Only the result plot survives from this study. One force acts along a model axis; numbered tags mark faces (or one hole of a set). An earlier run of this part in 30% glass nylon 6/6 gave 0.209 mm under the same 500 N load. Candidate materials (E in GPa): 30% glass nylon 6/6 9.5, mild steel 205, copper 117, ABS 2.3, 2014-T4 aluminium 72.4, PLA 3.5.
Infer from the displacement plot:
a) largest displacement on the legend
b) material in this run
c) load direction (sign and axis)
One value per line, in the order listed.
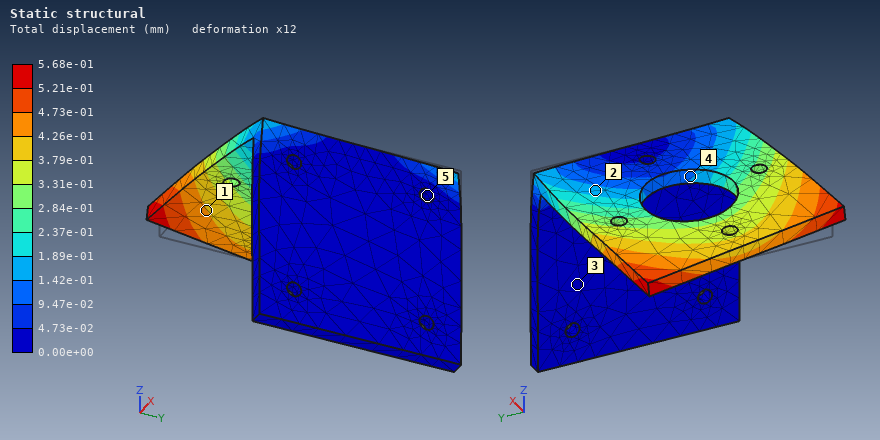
5.68e-01 mm
PLA
-Y
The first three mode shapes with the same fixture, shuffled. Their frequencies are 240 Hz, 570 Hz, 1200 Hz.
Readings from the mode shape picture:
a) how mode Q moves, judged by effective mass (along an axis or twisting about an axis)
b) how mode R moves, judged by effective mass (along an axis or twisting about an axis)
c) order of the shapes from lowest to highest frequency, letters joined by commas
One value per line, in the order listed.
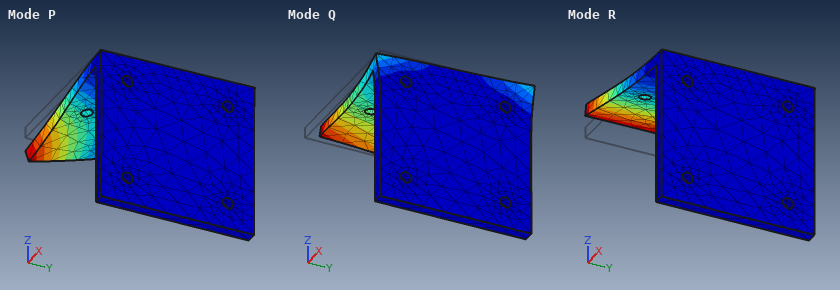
along Y
along Z
R, P, Q
